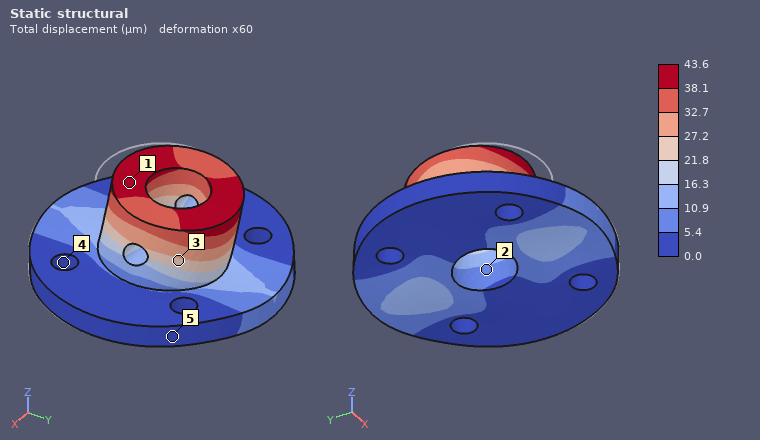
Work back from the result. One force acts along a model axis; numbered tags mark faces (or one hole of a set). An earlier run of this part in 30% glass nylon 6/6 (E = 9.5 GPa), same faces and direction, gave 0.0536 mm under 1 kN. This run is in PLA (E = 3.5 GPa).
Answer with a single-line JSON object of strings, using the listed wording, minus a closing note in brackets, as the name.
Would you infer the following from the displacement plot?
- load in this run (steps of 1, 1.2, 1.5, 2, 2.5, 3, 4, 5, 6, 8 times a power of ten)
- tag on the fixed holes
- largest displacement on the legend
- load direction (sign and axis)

{"load in this run": "300 N", "tag on the fixed holes": "4", "largest displacement on the legend": "43.6 µm", "load direction": "+Y"}
